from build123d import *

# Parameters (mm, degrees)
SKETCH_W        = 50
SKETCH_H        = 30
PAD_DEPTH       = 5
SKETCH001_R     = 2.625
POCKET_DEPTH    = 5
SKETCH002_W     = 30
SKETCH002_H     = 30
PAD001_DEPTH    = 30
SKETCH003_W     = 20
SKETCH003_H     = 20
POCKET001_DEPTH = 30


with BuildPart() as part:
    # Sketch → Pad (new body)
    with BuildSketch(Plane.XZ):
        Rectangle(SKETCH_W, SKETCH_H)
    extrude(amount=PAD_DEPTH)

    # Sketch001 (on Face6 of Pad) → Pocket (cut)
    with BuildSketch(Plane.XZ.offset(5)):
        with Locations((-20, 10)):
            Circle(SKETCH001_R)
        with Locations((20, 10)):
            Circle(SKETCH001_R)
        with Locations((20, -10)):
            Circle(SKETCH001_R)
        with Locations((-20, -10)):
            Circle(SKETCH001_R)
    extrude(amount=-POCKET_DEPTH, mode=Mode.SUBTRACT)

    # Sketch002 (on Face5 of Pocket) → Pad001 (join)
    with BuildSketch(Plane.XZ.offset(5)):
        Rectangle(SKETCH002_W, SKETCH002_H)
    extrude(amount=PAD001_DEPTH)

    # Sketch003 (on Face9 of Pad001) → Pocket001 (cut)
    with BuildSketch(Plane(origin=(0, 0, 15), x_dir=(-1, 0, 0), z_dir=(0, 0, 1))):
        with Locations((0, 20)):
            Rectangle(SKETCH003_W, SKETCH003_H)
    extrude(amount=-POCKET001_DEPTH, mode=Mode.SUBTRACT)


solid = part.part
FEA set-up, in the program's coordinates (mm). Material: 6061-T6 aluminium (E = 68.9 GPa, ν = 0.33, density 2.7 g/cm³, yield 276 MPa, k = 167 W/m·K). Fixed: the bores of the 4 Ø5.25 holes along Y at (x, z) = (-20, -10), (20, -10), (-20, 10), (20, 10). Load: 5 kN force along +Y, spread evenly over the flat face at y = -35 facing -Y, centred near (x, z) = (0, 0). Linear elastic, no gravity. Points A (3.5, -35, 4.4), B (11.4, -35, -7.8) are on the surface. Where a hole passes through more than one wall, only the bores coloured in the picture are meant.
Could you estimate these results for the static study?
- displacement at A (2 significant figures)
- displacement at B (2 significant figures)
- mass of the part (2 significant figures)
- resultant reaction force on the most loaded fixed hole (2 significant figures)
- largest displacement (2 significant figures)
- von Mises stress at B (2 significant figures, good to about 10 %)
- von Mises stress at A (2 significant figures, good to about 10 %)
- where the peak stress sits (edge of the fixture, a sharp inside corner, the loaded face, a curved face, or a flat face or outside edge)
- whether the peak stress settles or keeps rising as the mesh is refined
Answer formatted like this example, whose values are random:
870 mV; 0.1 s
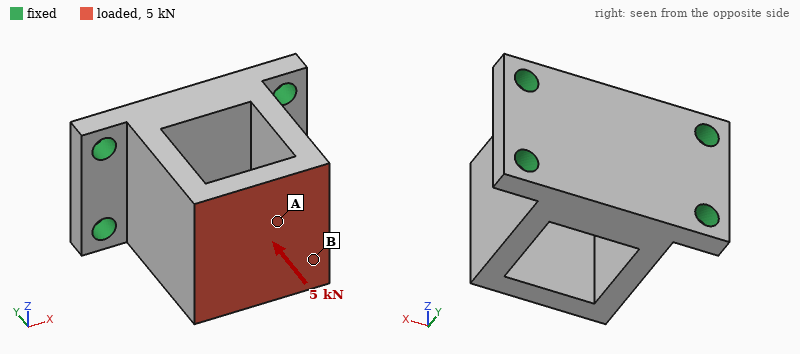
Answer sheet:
27 µm; 16 µm; 60 g; 1.3 kN; 32 µm; 13 MPa; 37 MPa; edge of the fixture; keeps rising
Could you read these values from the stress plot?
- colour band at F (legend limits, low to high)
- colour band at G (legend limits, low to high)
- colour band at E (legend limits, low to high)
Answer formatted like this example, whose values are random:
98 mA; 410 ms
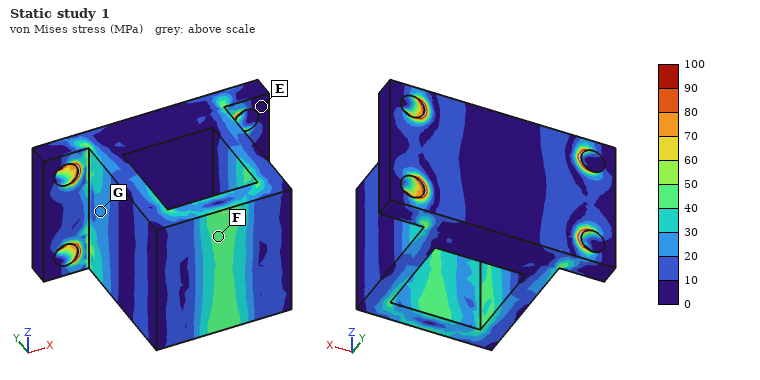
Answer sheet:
40 to 50 MPa; 20 to 30 MPa; 0 to 10 MPa
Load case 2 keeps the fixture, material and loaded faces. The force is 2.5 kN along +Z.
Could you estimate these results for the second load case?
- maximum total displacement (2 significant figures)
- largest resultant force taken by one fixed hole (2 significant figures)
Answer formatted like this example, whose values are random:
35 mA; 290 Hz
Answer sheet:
72 µm; 2.1 kN
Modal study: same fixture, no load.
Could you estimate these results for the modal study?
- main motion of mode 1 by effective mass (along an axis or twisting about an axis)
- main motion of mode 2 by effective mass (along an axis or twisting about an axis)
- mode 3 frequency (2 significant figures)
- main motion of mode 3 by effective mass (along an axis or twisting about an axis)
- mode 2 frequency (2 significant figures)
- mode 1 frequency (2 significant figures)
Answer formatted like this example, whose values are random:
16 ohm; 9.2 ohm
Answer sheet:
along X; along Z; 12 kHz; twisting about Y; 7500 Hz; 5700 Hz
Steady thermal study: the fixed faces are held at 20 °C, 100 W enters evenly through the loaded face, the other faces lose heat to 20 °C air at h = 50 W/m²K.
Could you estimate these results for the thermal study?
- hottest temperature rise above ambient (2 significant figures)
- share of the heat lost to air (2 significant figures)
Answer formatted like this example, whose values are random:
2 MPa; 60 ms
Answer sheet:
69 K; 11 %
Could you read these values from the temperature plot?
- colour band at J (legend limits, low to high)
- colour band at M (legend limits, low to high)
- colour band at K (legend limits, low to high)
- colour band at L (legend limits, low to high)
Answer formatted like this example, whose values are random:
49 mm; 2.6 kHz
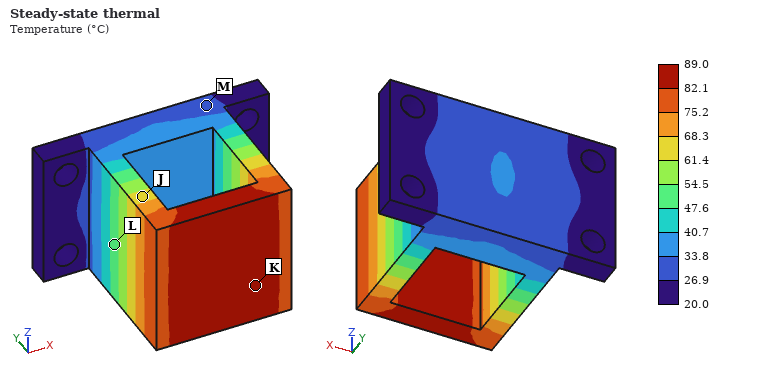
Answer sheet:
61.4 to 68.3 °C; 26.9 to 33.8 °C; 82.1 to 89.0 °C; 47.6 to 54.5 °C
